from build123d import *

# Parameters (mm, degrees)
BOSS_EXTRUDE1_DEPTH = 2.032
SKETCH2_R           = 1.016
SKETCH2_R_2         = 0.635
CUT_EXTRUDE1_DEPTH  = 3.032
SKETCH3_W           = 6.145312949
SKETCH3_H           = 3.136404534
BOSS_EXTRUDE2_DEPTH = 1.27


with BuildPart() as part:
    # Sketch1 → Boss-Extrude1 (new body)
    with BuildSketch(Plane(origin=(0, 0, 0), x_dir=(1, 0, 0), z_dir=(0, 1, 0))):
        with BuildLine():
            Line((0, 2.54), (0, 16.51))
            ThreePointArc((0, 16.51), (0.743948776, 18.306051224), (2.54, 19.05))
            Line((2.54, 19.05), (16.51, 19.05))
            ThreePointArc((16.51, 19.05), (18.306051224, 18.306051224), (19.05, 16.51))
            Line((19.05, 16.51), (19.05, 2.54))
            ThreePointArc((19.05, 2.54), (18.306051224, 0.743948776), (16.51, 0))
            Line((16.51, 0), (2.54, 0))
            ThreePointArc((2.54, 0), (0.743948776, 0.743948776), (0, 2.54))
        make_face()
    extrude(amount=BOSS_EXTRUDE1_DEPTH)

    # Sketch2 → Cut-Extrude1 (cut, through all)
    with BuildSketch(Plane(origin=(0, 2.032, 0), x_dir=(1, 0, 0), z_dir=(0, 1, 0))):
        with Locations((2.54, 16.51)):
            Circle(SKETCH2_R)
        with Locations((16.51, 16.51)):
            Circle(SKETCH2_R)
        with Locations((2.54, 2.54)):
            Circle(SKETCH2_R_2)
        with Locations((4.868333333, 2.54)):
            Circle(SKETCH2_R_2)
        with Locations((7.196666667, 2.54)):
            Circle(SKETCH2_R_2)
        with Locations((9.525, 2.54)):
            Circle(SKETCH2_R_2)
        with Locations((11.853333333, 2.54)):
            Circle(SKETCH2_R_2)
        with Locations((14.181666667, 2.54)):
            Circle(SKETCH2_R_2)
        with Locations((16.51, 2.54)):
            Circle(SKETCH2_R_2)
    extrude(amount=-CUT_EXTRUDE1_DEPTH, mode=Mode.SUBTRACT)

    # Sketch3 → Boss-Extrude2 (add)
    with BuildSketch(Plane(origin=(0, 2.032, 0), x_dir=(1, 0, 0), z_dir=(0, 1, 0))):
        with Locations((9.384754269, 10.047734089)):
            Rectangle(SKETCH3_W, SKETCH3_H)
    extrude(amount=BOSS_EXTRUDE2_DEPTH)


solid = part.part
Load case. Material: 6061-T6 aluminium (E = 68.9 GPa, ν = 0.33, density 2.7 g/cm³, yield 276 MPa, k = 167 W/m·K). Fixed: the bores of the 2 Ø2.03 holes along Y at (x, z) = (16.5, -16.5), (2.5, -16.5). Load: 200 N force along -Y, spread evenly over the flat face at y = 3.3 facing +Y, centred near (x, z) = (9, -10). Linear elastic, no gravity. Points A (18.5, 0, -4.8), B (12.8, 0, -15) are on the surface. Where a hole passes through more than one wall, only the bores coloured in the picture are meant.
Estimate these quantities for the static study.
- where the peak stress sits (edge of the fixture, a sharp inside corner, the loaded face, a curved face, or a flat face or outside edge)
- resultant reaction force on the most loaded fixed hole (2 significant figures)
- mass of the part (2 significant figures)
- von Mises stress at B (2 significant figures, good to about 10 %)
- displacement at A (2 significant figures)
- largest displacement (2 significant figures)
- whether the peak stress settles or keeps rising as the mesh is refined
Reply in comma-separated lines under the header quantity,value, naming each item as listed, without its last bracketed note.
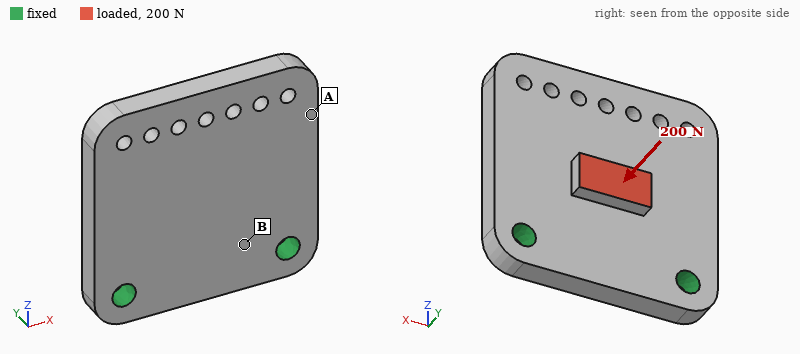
quantity,value
where the peak stress sits,edge of the fixture
resultant reaction force on the most loaded fixed hole,100 N
mass of the part,1.9 g
von Mises stress at B,48 MPa
displacement at A,50 µm
largest displacement,86 µm
whether the peak stress settles or keeps rising as the mesh is refined,keeps rising
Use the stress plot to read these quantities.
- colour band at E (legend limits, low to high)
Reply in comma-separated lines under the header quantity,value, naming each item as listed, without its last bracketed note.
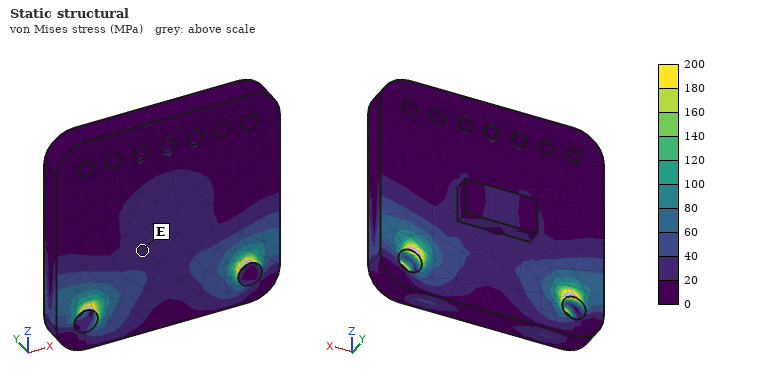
quantity,value
colour band at E,20 to 40 MPa
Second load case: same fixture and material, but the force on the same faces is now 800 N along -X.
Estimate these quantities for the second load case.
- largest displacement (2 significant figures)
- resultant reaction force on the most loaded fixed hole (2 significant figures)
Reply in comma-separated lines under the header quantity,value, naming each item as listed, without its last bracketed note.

quantity,value
largest displacement,35 µm
resultant reaction force on the most loaded fixed hole,540 N
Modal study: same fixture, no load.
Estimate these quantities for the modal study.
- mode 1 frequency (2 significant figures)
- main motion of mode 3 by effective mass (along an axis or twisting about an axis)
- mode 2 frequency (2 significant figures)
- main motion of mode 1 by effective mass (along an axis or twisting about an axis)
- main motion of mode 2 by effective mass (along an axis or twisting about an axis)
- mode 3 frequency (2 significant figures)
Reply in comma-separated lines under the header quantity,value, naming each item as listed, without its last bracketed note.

quantity,value
mode 1 frequency,6100 Hz
main motion of mode 3 by effective mass,along Y
mode 2 frequency,14 kHz
main motion of mode 1 by effective mass,along Y
main motion of mode 2 by effective mass,twisting about Z
mode 3 frequency,34 kHz
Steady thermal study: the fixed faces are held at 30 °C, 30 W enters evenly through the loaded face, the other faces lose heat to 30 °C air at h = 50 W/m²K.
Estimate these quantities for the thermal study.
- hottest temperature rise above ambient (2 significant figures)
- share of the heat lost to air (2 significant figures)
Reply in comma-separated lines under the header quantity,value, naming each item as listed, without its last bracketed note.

quantity,value
hottest temperature rise above ambient,59 K
share of the heat lost to air,3.9 %
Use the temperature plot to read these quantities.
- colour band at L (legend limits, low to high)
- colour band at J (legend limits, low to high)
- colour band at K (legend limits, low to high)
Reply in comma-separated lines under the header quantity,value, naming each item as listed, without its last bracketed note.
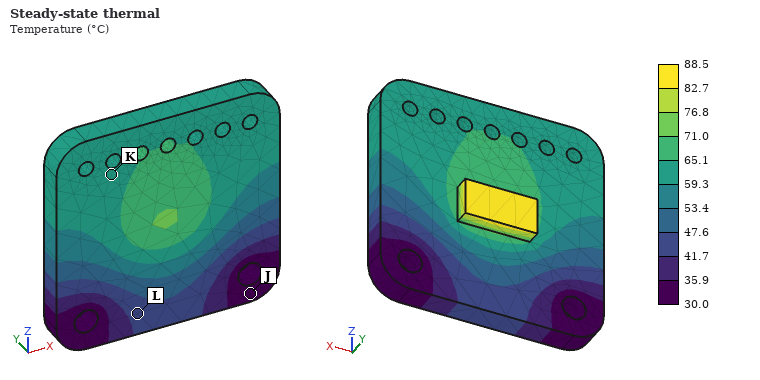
quantity,value
colour band at L,41.7 to 47.6 °C
colour band at J,30.0 to 35.9 °C
colour band at K,59.3 to 65.1 °C
